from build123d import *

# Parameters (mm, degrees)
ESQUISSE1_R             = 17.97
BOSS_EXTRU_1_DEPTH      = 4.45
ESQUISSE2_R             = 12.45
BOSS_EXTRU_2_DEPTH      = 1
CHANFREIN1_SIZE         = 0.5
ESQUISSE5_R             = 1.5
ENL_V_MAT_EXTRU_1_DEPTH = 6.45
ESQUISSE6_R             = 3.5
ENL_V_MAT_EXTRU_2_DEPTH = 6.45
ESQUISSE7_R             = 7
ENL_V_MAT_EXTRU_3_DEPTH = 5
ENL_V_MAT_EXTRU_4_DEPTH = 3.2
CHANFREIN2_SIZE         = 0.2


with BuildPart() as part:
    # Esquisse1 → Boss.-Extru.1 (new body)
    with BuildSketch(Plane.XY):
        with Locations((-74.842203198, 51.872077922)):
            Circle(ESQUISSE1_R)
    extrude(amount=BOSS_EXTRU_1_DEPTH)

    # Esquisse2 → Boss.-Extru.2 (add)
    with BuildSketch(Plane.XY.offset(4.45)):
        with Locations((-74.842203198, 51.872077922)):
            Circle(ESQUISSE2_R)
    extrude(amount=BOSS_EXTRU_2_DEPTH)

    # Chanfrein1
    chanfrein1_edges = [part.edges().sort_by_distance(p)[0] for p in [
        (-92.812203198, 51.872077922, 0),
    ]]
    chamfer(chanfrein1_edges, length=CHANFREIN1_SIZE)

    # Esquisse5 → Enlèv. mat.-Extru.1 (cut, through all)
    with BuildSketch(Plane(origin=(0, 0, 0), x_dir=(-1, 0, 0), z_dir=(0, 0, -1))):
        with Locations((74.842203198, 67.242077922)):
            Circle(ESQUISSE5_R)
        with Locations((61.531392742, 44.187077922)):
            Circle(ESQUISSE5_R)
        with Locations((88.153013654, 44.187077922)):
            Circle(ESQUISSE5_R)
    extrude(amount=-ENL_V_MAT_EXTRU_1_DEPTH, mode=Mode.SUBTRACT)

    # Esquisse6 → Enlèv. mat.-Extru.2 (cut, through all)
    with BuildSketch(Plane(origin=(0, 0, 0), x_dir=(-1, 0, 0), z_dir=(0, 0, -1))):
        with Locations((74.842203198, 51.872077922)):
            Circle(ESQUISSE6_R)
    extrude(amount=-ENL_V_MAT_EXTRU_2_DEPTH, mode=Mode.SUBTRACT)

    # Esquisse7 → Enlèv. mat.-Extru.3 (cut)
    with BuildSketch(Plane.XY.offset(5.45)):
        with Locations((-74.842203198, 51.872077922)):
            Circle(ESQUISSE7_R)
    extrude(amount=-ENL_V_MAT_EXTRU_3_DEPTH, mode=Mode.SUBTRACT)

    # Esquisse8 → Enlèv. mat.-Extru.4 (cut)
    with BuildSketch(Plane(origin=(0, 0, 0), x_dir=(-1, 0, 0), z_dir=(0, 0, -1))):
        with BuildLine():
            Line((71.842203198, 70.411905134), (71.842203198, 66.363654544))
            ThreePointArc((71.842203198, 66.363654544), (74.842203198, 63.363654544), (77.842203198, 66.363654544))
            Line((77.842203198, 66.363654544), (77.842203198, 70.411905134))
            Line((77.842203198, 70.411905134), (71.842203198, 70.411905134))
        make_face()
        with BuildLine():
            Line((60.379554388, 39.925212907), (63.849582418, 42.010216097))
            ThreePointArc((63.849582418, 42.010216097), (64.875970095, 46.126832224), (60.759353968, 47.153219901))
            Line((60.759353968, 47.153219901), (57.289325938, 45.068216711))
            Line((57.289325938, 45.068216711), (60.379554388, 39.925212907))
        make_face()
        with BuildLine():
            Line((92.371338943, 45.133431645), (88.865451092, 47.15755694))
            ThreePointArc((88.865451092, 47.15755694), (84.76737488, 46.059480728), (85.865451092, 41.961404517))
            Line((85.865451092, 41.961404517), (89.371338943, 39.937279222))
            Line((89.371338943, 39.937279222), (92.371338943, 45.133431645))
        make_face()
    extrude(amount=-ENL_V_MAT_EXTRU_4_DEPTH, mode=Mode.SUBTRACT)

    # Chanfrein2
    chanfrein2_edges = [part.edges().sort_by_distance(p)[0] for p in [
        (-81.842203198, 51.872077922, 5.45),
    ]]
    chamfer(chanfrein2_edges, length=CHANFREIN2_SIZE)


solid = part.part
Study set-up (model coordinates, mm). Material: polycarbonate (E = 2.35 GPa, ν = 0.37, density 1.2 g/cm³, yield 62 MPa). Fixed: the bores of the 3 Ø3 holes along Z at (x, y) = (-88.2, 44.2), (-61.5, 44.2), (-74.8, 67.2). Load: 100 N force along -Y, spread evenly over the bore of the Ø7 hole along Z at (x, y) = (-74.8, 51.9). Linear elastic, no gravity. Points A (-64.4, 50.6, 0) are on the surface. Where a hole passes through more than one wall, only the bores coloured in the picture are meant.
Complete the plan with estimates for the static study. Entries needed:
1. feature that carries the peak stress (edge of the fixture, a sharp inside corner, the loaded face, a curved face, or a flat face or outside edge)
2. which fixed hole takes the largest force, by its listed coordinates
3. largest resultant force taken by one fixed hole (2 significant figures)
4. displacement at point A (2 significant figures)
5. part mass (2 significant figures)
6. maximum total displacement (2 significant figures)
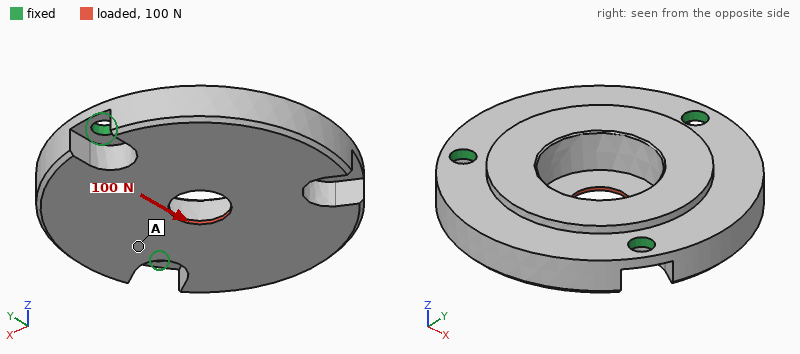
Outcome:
the loaded face
(-74.8, 67.2)
41 N
12 µm
4.6 g
44 µm
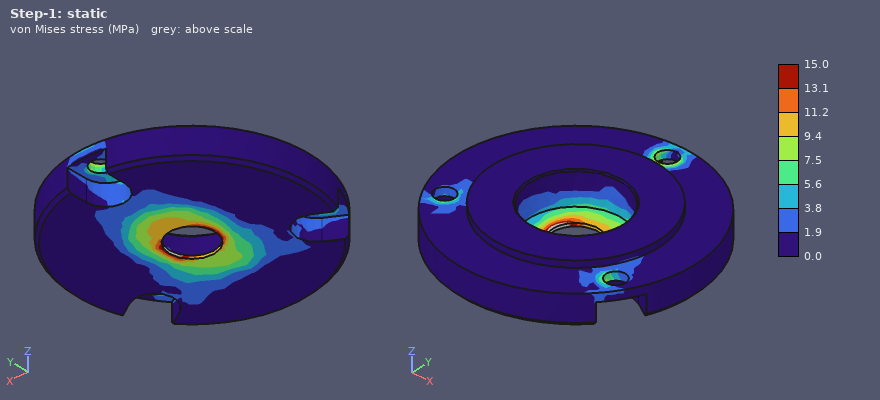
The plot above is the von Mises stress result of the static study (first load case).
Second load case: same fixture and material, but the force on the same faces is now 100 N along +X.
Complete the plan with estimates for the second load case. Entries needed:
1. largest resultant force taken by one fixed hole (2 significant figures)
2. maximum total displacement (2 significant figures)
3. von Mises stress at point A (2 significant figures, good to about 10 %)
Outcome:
38 N
40 µm
2.6 MPa
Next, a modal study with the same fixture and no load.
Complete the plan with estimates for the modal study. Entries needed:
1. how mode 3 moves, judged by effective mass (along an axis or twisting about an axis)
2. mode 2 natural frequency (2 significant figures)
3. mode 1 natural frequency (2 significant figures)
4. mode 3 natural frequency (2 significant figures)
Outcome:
along Z
3600 Hz
3600 Hz
4500 Hz
